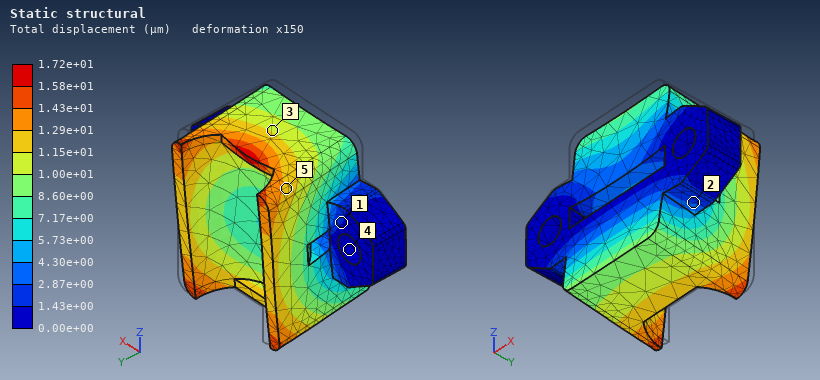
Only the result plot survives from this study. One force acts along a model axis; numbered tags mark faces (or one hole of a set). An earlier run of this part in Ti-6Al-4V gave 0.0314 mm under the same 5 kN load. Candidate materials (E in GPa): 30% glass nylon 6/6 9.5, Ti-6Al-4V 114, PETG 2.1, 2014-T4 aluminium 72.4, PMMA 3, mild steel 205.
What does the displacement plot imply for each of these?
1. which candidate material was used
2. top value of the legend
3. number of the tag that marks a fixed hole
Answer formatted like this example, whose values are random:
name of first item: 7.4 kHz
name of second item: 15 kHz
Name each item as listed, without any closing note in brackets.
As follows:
which candidate material was used: mild steel
top value of the legend: 1.72e+01 µm
number of the tag that marks a fixed hole: 4
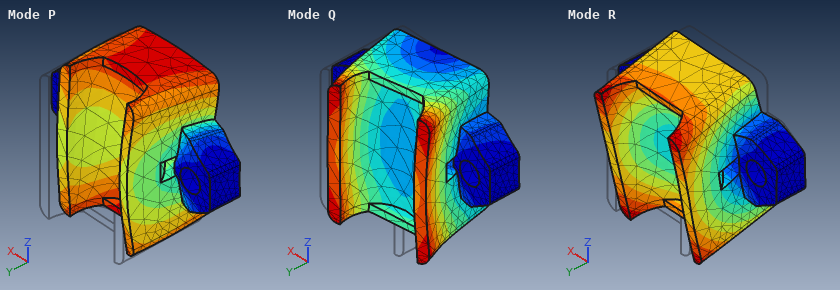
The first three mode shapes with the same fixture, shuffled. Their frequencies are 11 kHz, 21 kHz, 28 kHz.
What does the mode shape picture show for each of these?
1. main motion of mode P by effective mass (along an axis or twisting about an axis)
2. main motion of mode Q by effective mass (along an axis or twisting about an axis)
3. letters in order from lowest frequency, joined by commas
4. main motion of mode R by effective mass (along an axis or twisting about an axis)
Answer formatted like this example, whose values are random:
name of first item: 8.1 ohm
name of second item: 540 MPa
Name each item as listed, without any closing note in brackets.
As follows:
main motion of mode P by effective mass: along Y
main motion of mode Q by effective mass: along X
letters in order from lowest frequency, joined by commas: R, P, Q
main motion of mode R by effective mass: along Z
